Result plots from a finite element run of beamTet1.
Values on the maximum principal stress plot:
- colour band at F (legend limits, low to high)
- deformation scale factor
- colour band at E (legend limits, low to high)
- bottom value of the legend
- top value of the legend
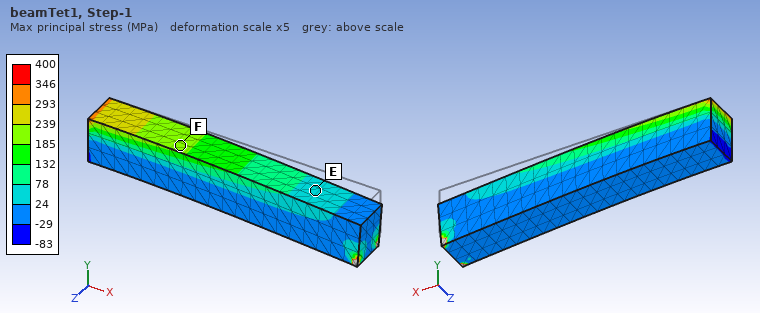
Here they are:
185 to 239 MPa
5
24 to 78 MPa
-83 MPa
400 MPa
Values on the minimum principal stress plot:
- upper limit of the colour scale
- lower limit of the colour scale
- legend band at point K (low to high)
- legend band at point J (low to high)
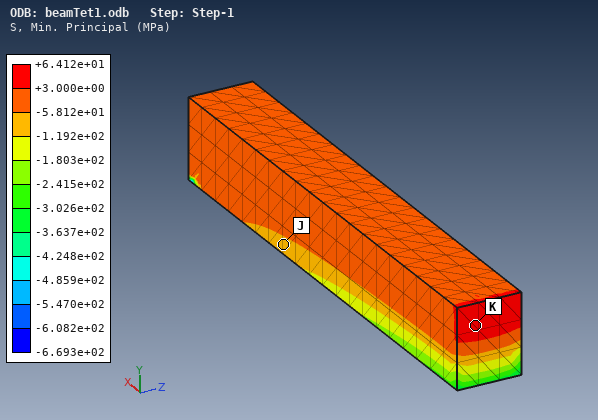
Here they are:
+6.412e+01 MPa
-6.693e+02 MPa
+3.000e+00 to +6.412e+01 MPa
-1.192e+02 to -5.812e+01 MPa
